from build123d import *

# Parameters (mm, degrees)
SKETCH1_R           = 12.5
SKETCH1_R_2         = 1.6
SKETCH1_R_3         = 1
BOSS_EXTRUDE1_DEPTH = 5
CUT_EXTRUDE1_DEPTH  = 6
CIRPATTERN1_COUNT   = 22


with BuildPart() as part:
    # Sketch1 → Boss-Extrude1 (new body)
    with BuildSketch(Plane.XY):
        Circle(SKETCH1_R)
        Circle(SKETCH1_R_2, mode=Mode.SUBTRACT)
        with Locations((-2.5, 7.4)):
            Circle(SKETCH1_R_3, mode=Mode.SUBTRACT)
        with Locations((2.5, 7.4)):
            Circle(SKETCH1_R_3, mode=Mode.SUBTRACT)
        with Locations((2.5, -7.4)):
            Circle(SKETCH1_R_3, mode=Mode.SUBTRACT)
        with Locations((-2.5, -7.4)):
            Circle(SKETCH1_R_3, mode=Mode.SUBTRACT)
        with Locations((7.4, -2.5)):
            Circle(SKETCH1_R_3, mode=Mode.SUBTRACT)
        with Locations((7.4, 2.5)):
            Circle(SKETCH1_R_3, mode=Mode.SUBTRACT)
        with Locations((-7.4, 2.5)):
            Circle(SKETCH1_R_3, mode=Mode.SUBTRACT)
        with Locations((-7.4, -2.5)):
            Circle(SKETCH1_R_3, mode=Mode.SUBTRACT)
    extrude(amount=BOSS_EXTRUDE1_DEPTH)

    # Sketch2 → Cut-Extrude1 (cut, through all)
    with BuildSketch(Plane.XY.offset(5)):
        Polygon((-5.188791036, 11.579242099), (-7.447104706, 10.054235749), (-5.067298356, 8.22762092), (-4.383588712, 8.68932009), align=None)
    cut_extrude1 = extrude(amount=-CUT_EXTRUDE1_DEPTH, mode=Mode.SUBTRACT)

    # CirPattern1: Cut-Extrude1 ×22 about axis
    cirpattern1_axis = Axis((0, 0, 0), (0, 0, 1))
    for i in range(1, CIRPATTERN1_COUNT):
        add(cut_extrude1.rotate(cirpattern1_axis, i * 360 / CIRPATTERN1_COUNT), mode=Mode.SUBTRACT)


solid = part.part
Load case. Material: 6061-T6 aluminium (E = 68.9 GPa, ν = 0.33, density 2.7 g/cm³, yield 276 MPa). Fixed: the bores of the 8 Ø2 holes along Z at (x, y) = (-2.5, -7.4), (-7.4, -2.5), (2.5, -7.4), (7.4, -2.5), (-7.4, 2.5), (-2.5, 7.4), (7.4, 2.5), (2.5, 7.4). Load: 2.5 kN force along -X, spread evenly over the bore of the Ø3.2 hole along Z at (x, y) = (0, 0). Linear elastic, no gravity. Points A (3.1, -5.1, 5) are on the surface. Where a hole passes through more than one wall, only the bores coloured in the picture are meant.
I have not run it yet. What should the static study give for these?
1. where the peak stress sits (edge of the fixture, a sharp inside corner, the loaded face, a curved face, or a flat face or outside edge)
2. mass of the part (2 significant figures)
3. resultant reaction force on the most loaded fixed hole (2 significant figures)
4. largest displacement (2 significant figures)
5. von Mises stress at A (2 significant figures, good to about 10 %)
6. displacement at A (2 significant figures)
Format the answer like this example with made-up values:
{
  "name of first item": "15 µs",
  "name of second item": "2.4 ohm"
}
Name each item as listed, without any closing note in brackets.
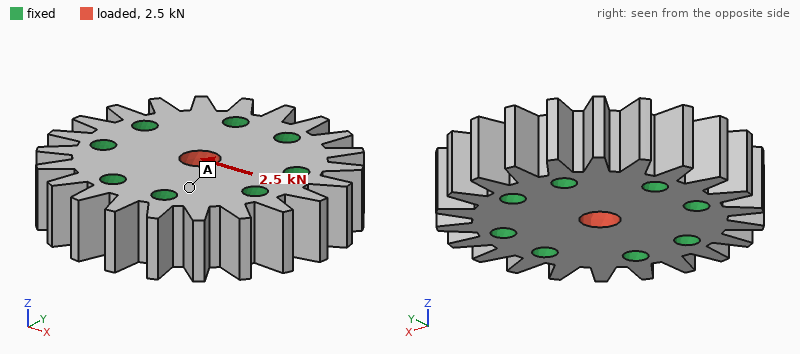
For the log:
{
  "where the peak stress sits": "the loaded face",
  "mass of the part": "4.7 g",
  "resultant reaction force on the most loaded fixed hole": "520 N",
  "largest displacement": "3.0 µm",
  "von Mises stress at A": "10 MPa",
  "displacement at A": "0.53 µm"
}
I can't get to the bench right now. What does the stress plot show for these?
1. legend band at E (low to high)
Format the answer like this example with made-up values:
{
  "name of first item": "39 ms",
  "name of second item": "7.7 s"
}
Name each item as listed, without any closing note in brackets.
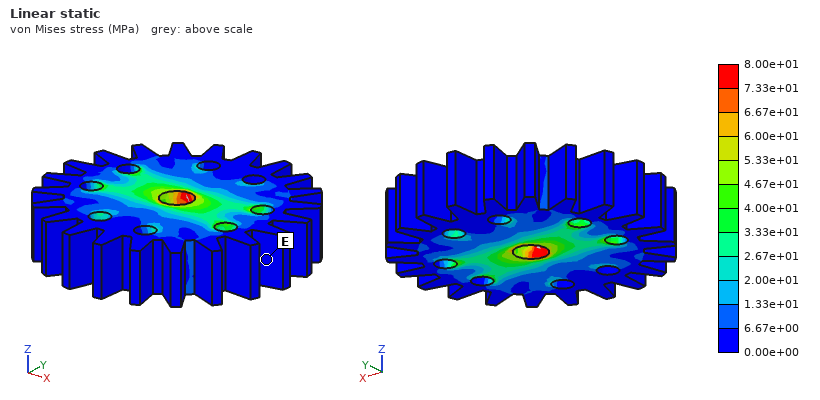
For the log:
{
  "legend band at E": "0.00e+00 to 6.67e+00 MPa"
}
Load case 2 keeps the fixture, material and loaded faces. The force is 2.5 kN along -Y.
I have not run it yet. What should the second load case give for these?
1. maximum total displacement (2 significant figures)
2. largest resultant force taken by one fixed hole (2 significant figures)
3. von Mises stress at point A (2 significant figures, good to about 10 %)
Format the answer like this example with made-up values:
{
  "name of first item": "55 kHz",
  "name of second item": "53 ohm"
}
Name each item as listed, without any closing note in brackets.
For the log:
{
  "maximum total displacement": "2.9 µm",
  "largest resultant force taken by one fixed hole": "520 N",
  "von Mises stress at point A": "19 MPa"
}
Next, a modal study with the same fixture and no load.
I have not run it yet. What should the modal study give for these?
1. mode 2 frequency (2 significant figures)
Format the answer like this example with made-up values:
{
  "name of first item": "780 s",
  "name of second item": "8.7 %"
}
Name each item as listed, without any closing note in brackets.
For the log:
{
  "mode 2 frequency": "120 kHz"
}
